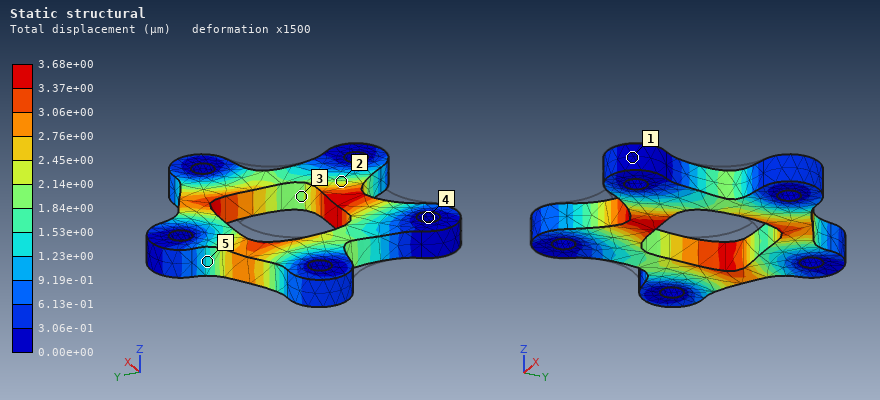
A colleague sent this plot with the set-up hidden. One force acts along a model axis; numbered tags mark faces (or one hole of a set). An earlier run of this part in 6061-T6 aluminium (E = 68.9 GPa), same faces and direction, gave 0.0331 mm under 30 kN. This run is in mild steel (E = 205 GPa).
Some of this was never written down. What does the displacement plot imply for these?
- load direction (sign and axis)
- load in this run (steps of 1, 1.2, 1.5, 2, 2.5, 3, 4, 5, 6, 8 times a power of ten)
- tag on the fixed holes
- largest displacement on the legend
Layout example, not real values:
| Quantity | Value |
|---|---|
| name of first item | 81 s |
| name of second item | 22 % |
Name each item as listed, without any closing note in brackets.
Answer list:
| Quantity | Value |
|---|---|
| load direction | +Y |
| load in this run | 10 kN |
| tag on the fixed holes | 4 |
| largest displacement on the legend | 3.68e+00 µm |
